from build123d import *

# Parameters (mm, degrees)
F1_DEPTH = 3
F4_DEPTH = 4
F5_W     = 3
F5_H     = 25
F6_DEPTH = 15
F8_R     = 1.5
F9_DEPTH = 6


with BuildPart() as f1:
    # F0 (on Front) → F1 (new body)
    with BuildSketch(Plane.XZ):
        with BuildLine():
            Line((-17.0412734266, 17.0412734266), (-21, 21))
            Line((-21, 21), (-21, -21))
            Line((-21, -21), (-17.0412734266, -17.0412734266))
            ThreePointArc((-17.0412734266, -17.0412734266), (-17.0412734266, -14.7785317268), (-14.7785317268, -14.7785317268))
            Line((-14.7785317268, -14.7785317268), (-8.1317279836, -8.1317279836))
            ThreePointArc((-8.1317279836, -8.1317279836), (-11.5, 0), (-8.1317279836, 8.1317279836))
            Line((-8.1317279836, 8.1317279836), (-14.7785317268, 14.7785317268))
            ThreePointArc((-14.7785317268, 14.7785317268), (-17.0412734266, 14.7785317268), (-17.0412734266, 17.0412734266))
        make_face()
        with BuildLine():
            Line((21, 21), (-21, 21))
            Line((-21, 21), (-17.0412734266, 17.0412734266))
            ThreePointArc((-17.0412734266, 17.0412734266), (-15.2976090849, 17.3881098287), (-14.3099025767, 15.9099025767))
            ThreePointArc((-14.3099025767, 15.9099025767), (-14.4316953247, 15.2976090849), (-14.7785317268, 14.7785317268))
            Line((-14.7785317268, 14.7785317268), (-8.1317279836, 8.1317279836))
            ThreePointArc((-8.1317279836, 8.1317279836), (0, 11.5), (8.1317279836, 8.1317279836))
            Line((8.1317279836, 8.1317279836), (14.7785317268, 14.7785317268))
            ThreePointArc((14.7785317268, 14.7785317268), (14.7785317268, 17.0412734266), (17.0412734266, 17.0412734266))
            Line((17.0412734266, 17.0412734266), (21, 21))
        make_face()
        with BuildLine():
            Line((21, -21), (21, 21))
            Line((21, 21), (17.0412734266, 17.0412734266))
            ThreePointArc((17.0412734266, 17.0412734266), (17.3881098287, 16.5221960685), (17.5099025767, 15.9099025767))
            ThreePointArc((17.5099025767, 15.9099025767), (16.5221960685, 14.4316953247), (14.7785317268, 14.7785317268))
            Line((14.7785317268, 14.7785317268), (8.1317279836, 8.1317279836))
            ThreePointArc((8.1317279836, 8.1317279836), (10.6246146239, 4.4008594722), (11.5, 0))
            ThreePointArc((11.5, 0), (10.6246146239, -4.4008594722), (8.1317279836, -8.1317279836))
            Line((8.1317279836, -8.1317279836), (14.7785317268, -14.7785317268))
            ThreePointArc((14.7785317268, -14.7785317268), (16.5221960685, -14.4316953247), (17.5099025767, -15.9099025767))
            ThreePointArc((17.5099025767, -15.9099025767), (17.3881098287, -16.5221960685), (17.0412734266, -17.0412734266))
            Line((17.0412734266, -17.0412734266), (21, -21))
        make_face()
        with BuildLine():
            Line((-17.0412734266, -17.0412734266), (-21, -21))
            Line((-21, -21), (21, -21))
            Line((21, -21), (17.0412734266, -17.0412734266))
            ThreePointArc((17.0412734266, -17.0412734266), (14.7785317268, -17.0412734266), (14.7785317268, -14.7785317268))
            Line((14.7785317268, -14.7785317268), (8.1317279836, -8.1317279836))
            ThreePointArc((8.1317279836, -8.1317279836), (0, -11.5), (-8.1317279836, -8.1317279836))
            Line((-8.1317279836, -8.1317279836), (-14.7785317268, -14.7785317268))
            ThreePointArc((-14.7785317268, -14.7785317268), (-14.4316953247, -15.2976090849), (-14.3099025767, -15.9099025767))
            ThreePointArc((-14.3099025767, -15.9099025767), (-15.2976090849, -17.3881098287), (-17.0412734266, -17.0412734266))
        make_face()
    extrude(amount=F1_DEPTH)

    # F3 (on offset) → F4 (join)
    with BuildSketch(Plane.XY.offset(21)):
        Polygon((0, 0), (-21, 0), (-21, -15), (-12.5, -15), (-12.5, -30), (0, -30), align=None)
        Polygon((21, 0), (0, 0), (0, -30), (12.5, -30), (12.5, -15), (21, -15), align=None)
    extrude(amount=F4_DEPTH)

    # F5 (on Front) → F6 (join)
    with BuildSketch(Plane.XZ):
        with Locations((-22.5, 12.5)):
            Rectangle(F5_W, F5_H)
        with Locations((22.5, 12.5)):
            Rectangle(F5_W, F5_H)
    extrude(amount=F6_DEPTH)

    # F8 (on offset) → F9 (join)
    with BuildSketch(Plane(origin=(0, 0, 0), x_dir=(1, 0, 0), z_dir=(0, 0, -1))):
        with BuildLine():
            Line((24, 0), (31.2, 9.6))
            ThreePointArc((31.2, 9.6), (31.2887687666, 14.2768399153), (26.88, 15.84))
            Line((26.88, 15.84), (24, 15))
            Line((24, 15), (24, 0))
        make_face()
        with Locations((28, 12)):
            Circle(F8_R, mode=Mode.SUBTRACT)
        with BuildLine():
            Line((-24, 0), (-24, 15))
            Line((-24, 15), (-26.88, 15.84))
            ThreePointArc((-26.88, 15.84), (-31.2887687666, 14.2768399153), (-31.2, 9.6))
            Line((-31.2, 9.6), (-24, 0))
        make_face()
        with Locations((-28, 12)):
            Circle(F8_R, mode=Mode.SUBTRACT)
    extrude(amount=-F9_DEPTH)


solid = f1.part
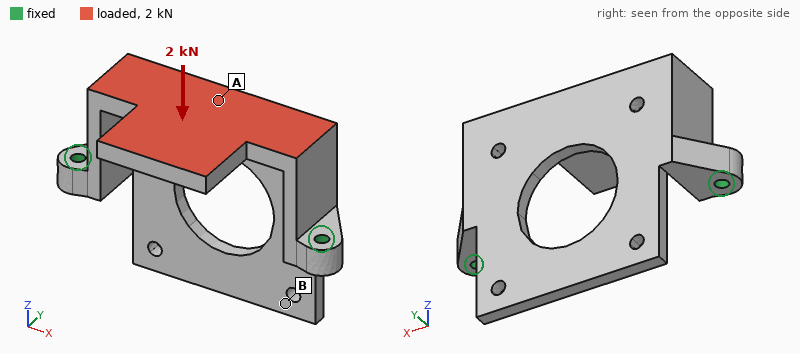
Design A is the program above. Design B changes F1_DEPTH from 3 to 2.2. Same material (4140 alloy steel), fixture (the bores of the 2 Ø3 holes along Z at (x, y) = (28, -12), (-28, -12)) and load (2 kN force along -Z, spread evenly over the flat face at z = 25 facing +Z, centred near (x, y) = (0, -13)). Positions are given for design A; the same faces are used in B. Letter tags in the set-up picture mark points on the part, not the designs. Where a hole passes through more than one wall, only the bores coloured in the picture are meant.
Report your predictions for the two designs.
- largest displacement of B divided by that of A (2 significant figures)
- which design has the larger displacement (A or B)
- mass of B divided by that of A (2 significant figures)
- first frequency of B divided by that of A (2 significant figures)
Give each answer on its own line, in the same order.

1.1
B
0.91
0.79
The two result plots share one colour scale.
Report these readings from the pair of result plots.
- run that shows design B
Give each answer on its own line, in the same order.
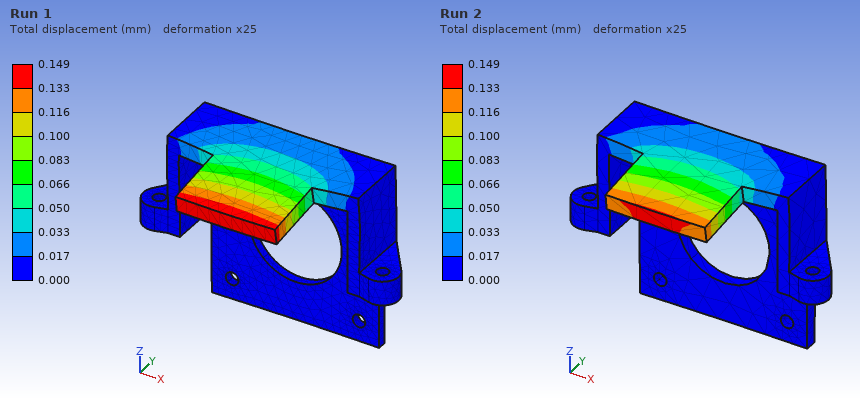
Run 1
